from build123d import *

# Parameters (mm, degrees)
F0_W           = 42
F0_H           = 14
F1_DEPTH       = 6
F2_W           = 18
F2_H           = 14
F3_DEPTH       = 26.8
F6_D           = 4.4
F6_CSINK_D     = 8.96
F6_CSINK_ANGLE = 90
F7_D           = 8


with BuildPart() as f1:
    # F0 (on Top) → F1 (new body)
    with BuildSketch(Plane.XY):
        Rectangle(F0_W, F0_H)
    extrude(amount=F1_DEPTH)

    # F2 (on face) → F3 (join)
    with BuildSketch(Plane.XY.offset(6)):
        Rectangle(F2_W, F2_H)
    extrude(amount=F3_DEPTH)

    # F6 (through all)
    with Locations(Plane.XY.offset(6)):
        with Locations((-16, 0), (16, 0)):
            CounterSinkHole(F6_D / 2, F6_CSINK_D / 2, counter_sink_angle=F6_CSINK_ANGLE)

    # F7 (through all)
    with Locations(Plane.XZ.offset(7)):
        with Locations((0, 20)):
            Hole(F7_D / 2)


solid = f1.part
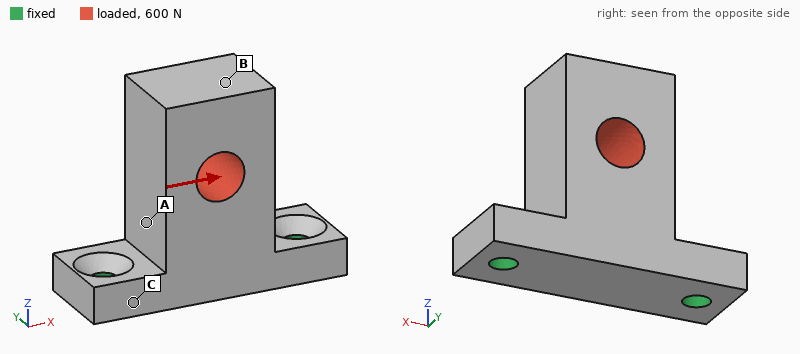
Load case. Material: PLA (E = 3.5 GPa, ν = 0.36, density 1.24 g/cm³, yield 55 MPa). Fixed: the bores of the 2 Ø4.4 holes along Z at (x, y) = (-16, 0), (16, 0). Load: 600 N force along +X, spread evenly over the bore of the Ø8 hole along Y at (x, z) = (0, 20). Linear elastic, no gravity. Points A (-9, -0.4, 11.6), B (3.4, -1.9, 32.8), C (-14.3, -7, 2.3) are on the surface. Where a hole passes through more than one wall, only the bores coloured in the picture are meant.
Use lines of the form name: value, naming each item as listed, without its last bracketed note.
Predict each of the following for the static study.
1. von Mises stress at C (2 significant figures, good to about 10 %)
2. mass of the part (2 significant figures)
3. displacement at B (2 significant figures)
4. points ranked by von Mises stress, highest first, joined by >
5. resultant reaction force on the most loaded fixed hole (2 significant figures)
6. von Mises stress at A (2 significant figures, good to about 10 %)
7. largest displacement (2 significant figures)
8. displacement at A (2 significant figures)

von Mises stress at C: 5.5 MPa
mass of the part: 12 g
displacement at B: 0.29 mm
points ranked by von Mises stress, highest first, joined by >: A > C > B
resultant reaction force on the most loaded fixed hole: 500 N
von Mises stress at A: 8.7 MPa
largest displacement: 0.30 mm
displacement at A: 0.10 mm
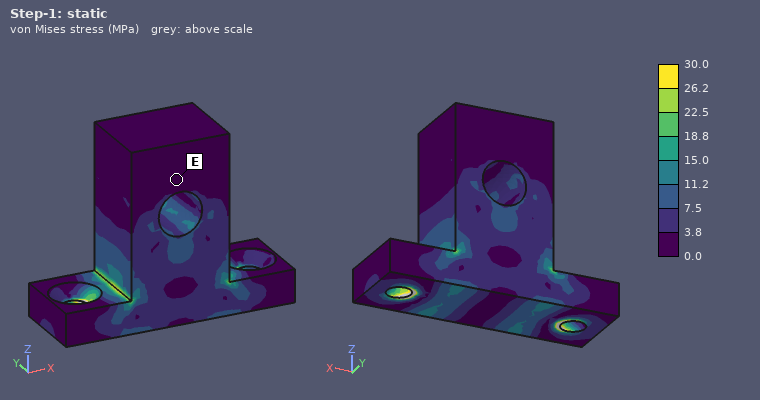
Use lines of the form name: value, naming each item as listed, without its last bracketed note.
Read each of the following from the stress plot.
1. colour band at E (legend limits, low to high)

colour band at E: 0.0 to 3.8 MPa
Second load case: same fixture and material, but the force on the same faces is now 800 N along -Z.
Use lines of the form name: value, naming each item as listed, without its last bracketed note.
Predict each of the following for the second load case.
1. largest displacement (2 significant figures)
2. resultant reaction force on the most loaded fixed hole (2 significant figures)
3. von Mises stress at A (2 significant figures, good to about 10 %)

largest displacement: 0.10 mm
resultant reaction force on the most loaded fixed hole: 480 N
von Mises stress at A: 5.0 MPa
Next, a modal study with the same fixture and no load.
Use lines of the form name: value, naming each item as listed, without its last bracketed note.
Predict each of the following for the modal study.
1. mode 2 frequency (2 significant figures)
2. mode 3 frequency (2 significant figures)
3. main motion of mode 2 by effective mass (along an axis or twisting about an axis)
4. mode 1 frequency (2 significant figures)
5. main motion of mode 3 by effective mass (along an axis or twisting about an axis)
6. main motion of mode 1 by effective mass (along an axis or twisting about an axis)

mode 2 frequency: 3000 Hz
mode 3 frequency: 4800 Hz
main motion of mode 2 by effective mass: along X
mode 1 frequency: 1200 Hz
main motion of mode 3 by effective mass: along Z
main motion of mode 1 by effective mass: along Y
